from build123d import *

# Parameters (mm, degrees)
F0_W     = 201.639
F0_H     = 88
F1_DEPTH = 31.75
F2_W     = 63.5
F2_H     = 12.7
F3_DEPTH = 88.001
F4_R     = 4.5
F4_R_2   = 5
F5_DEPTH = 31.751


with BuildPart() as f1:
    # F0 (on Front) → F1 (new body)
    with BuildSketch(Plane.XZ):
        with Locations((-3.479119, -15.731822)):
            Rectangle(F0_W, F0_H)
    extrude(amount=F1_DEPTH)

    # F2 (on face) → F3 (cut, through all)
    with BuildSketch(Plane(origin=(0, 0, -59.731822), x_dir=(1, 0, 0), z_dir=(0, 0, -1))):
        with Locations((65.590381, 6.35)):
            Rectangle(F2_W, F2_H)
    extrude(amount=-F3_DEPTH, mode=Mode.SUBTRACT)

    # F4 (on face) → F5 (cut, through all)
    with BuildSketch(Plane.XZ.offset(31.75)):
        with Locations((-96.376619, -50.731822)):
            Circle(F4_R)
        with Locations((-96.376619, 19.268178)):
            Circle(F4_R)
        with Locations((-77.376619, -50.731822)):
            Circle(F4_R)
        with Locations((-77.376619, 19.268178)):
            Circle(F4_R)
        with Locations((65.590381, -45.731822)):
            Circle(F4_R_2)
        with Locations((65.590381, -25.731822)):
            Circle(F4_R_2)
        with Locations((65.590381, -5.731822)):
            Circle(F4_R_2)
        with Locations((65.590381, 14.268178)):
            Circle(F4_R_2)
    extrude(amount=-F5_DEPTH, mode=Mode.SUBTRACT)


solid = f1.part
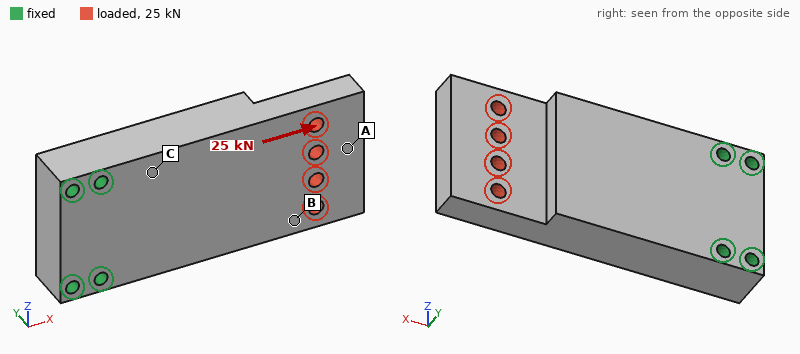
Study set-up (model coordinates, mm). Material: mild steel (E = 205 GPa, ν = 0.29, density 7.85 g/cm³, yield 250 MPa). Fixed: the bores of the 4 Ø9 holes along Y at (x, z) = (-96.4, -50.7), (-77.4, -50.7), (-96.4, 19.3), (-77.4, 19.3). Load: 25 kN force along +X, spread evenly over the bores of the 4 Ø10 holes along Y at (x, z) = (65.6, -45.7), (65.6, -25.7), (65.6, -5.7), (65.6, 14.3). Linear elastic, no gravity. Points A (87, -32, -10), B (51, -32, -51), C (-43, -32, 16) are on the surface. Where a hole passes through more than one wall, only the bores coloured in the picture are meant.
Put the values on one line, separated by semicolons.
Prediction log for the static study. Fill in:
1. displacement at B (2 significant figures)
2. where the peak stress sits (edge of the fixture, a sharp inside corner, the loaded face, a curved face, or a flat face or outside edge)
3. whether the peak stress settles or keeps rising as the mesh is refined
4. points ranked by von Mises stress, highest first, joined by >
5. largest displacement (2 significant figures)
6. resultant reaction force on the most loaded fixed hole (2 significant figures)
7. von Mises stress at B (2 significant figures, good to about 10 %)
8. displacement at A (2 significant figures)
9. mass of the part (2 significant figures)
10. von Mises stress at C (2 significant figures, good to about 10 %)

31 µm; edge of the fixture; keeps rising; C > B > A; 48 µm; 10 kN; 14 MPa; 45 µm; 3.8 kg; 21 MPa
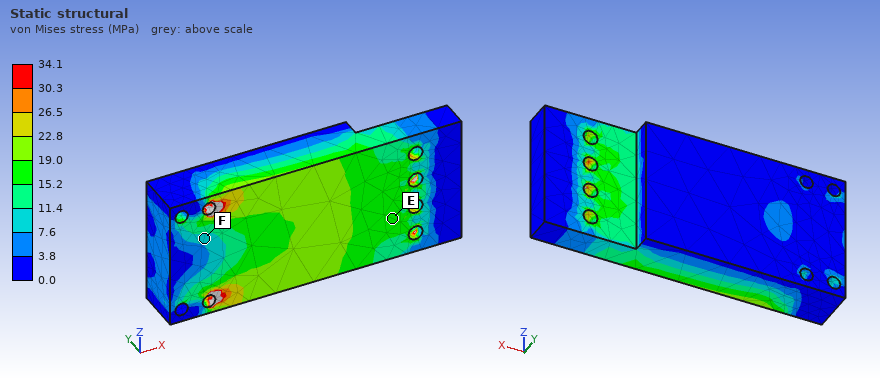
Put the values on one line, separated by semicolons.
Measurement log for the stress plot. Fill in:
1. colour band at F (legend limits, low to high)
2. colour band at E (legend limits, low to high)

7.6 to 11.4 MPa; 15.2 to 19.0 MPa
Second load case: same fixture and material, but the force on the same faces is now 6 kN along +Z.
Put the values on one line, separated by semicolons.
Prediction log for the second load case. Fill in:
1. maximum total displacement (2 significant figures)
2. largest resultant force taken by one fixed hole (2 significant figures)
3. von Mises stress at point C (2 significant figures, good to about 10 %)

29 µm; 11 kN; 12 MPa
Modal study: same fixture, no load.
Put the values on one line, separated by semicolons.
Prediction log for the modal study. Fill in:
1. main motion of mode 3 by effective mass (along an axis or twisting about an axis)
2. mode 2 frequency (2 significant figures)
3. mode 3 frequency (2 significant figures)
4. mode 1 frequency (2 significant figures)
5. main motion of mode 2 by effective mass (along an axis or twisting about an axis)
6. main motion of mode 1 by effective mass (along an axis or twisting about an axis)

twisting about X; 2500 Hz; 3200 Hz; 960 Hz; along Z; along Y
